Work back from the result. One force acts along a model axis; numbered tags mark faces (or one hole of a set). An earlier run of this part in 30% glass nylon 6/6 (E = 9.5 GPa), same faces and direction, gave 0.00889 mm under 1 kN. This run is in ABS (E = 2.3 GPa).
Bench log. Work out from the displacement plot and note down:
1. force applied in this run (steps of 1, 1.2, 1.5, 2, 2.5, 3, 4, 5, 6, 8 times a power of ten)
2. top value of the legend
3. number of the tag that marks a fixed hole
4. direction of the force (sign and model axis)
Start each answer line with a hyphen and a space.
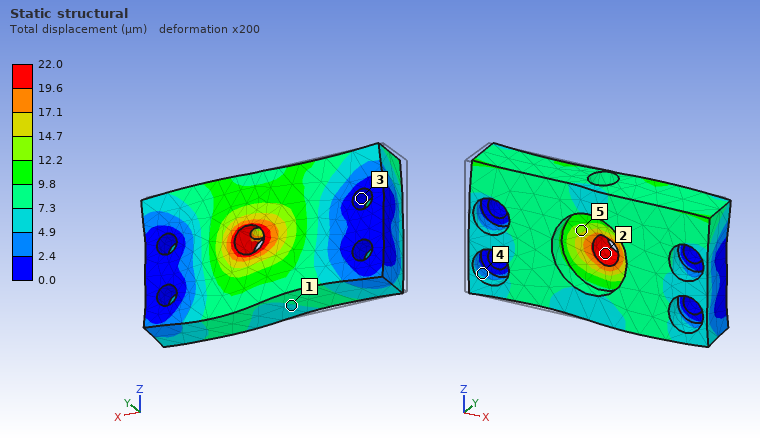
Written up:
- 600 N
- 22.0 µm
- 3
- +X
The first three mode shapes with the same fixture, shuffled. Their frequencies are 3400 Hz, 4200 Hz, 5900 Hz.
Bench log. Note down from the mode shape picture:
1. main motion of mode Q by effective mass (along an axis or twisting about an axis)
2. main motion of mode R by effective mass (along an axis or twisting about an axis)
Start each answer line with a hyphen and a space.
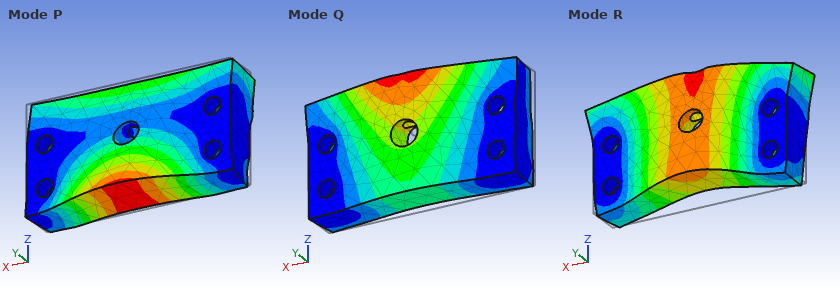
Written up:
- along Y
- along Z
